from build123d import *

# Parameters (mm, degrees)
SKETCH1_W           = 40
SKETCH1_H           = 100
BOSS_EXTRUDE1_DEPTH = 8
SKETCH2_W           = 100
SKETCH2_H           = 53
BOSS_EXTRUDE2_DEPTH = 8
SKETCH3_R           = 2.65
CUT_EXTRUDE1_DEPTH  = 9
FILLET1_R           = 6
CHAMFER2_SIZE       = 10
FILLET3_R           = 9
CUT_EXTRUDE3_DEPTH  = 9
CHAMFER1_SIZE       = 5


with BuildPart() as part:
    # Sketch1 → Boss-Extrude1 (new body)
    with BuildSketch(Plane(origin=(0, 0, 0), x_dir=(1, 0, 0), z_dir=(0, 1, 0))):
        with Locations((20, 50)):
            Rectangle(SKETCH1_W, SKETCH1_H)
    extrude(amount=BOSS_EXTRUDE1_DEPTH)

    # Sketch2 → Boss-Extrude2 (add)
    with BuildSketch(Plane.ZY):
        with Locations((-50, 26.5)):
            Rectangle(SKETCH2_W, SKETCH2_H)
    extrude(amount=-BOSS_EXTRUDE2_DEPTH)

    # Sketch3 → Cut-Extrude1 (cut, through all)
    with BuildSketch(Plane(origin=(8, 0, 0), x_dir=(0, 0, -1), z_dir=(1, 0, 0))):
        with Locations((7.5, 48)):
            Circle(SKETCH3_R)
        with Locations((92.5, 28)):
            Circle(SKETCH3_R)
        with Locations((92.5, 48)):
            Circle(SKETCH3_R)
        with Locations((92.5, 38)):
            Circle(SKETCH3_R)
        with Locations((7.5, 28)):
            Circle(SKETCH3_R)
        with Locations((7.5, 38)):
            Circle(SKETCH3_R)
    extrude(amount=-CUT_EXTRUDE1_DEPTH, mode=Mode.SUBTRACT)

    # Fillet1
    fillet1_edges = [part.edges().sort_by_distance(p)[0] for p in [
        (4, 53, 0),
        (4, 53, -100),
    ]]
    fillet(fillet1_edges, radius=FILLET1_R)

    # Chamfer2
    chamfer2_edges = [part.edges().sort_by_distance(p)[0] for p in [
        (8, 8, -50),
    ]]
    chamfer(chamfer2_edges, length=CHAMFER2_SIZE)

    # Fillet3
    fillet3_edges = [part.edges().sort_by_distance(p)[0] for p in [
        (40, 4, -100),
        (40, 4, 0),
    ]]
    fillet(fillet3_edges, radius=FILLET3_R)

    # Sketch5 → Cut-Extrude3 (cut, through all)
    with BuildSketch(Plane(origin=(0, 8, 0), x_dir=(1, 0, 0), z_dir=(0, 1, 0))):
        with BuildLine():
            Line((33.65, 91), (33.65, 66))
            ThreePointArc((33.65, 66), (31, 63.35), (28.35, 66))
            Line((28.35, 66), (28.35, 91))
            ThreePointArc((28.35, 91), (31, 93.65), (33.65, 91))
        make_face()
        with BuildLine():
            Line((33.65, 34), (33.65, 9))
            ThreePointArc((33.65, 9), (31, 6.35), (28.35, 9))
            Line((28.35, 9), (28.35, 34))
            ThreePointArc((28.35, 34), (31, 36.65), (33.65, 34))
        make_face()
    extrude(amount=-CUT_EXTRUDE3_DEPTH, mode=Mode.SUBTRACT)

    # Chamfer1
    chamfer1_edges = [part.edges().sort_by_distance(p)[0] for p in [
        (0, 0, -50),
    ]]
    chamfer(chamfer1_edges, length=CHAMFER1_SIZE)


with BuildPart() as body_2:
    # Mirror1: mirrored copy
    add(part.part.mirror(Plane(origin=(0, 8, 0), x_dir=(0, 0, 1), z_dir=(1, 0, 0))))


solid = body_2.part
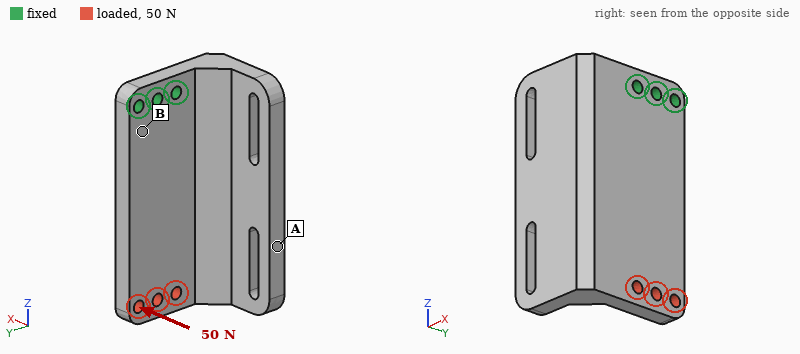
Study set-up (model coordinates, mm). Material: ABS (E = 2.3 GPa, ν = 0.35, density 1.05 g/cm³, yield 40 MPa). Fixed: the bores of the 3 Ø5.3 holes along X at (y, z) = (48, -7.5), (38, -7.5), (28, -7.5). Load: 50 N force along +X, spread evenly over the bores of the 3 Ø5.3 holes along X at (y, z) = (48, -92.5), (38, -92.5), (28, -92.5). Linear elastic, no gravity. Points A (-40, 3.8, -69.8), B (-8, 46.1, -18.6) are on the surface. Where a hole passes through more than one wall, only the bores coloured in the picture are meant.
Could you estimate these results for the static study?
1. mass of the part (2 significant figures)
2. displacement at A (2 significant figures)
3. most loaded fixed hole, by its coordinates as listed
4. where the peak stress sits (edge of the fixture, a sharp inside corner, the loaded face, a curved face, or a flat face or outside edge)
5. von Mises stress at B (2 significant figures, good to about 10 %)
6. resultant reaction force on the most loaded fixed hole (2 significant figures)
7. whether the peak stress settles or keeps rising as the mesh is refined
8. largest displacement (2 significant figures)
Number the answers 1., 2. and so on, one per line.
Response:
1. 71 g
2. 0.83 mm
3. (38, -7.5)
4. edge of the fixture
5. 5.5 MPa
6. 52 N
7. keeps rising
8. 1.3 mm
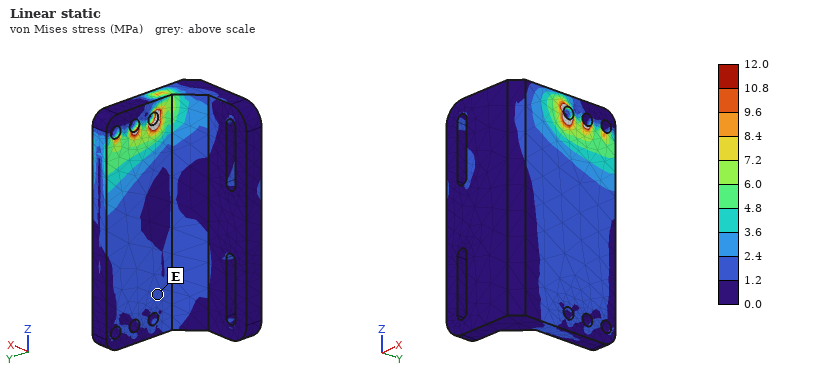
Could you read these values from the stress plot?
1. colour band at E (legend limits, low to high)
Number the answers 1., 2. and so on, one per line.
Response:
1. 1.2 to 2.4 MPa
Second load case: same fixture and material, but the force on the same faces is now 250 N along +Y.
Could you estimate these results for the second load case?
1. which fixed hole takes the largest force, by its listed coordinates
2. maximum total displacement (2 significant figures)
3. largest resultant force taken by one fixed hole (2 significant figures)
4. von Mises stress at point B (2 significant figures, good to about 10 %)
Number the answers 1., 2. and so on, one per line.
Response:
1. (28, -7.5)
2. 0.72 mm
3. 940 N
4. 7.4 MPa
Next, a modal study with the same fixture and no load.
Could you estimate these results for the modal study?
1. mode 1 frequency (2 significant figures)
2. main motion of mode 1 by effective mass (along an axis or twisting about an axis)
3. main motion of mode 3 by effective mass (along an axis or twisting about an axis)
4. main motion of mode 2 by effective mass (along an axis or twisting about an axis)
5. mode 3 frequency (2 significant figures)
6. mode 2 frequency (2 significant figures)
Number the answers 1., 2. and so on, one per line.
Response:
1. 210 Hz
2. along X
3. along Y
4. along Y
5. 670 Hz
6. 490 Hz
